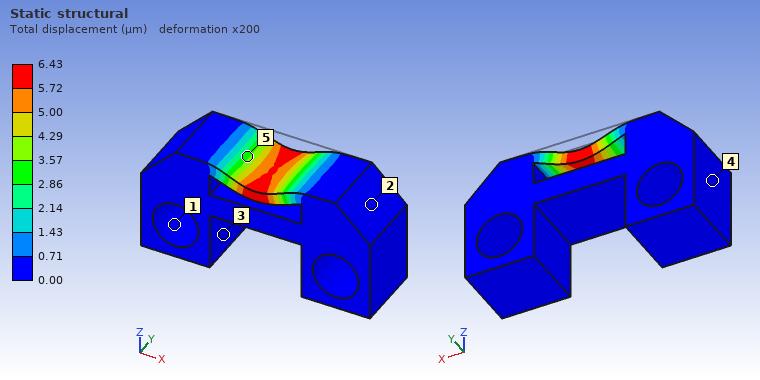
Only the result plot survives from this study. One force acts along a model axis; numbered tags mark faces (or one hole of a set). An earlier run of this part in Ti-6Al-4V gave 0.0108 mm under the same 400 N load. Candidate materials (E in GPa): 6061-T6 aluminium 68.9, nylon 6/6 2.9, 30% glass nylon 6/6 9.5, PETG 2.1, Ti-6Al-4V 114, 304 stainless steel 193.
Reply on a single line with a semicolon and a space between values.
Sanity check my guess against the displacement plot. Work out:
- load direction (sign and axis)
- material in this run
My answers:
-Z; 304 stainless steel
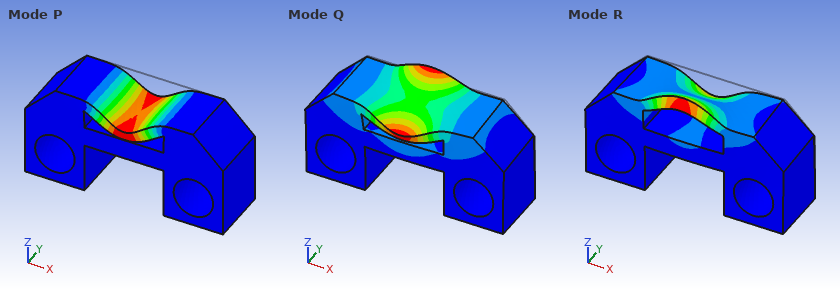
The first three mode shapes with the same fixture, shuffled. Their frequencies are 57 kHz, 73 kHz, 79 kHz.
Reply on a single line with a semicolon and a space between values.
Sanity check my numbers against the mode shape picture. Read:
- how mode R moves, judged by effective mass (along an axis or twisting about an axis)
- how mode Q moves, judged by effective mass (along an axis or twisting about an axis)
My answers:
along Y; along Y
